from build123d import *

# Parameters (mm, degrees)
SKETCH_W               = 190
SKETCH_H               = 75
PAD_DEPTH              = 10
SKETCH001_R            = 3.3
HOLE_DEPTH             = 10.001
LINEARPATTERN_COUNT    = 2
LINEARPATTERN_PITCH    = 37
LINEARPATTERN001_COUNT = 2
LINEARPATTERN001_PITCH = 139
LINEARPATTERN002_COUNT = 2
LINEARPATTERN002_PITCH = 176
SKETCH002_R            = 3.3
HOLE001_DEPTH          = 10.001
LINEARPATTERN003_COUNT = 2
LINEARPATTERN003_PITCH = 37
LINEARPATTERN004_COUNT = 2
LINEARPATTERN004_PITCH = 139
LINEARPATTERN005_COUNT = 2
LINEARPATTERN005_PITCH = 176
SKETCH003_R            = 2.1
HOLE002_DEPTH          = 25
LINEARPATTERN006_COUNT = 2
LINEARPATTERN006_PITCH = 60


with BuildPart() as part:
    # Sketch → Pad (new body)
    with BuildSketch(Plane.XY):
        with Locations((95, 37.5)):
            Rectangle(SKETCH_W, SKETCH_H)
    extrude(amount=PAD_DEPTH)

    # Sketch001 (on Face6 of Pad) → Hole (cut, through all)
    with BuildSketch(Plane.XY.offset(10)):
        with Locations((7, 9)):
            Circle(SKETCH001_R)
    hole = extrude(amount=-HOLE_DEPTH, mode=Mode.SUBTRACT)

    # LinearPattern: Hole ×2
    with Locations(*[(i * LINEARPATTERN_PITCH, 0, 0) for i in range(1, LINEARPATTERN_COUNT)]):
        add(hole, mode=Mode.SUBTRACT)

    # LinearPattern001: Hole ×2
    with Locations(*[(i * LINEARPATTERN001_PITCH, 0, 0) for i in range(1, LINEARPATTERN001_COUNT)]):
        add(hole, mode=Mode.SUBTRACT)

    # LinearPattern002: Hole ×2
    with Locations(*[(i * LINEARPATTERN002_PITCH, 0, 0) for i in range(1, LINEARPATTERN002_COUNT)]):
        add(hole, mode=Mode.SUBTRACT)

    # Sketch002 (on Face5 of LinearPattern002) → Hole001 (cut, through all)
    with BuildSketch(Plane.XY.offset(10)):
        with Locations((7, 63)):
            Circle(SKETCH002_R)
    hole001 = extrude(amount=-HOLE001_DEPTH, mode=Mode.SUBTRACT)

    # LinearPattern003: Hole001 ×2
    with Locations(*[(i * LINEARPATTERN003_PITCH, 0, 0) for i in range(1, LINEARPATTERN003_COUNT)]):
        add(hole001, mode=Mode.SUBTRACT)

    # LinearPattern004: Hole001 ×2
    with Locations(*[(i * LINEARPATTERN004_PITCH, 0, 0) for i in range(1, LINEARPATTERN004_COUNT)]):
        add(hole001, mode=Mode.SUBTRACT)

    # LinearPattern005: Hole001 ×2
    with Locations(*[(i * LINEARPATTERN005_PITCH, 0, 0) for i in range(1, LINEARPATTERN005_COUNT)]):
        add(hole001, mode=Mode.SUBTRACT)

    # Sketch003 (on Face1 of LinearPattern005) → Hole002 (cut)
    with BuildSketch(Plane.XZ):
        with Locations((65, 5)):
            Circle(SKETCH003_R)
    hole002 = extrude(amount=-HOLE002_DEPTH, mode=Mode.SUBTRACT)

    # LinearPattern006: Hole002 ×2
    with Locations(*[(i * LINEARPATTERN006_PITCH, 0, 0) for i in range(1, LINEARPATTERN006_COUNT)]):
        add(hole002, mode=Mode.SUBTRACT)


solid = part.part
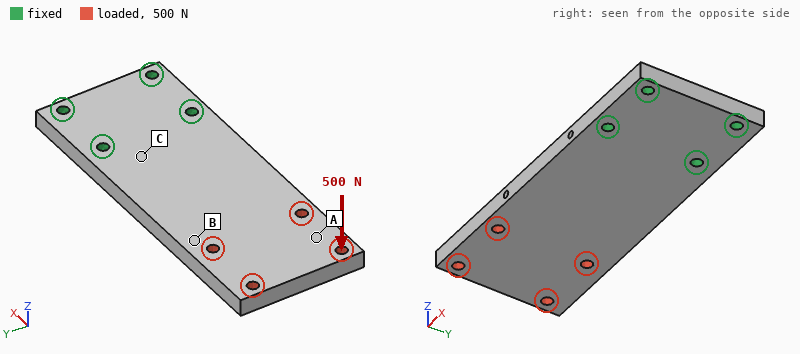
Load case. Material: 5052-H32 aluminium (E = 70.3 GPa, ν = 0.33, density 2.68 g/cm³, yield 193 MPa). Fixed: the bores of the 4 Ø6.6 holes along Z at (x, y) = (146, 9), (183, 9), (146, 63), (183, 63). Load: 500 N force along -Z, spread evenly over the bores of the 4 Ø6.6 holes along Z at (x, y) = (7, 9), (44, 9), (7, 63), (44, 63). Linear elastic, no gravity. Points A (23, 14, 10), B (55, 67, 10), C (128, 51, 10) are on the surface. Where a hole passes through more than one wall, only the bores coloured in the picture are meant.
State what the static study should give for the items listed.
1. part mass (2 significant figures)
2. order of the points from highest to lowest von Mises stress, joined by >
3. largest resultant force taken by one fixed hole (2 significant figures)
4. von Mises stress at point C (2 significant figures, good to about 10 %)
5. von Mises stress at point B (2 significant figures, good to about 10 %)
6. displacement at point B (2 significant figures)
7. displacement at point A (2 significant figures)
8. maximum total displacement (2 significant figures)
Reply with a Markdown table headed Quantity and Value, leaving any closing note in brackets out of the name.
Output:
| Quantity | Value |
|---|---|
| part mass | 370 g |
| order of the points from highest to lowest von Mises stress, joined by > | C > B > A |
| largest resultant force taken by one fixed hole | 560 N |
| von Mises stress at point C | 37 MPa |
| von Mises stress at point B | 12 MPa |
| displacement at point B | 0.44 mm |
| displacement at point A | 0.71 mm |
| maximum total displacement | 0.91 mm |
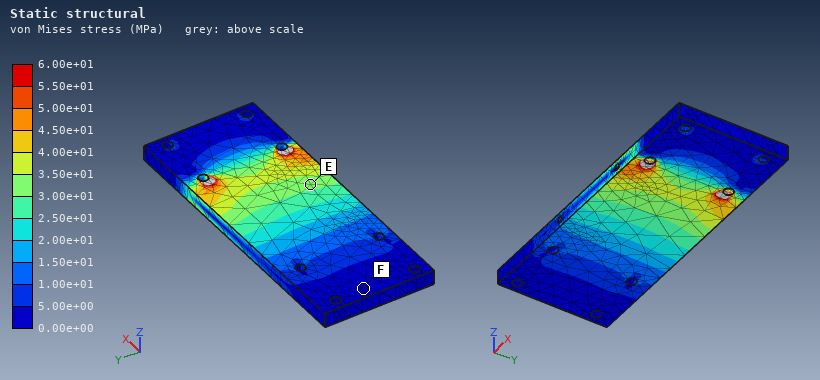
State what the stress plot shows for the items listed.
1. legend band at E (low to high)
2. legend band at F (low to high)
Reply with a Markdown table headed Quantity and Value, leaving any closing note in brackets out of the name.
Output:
| Quantity | Value |
|---|---|
| legend band at E | 3.00e+01 to 3.50e+01 MPa |
| legend band at F | 0.00e+00 to 5.00e+00 MPa |
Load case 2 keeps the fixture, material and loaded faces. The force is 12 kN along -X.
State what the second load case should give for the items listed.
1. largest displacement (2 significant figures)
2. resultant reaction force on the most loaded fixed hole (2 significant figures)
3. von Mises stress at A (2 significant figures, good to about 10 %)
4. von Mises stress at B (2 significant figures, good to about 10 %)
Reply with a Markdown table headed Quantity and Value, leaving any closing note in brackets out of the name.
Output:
| Quantity | Value |
|---|---|
| largest displacement | 42 µm |
| resultant reaction force on the most loaded fixed hole | 5.1 kN |
| von Mises stress at A | 12 MPa |
| von Mises stress at B | 18 MPa |
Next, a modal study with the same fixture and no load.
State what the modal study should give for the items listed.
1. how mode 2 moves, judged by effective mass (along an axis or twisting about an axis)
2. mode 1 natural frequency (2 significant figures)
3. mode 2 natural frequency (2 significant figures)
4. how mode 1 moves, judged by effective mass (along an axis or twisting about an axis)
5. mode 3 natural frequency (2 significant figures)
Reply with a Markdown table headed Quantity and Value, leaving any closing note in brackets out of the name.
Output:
| Quantity | Value |
|---|---|
| how mode 2 moves, judged by effective mass | twisting about X |
| mode 1 natural frequency | 390 Hz |
| mode 2 natural frequency | 1600 Hz |
| how mode 1 moves, judged by effective mass | along Z |
| mode 3 natural frequency | 2300 Hz |
